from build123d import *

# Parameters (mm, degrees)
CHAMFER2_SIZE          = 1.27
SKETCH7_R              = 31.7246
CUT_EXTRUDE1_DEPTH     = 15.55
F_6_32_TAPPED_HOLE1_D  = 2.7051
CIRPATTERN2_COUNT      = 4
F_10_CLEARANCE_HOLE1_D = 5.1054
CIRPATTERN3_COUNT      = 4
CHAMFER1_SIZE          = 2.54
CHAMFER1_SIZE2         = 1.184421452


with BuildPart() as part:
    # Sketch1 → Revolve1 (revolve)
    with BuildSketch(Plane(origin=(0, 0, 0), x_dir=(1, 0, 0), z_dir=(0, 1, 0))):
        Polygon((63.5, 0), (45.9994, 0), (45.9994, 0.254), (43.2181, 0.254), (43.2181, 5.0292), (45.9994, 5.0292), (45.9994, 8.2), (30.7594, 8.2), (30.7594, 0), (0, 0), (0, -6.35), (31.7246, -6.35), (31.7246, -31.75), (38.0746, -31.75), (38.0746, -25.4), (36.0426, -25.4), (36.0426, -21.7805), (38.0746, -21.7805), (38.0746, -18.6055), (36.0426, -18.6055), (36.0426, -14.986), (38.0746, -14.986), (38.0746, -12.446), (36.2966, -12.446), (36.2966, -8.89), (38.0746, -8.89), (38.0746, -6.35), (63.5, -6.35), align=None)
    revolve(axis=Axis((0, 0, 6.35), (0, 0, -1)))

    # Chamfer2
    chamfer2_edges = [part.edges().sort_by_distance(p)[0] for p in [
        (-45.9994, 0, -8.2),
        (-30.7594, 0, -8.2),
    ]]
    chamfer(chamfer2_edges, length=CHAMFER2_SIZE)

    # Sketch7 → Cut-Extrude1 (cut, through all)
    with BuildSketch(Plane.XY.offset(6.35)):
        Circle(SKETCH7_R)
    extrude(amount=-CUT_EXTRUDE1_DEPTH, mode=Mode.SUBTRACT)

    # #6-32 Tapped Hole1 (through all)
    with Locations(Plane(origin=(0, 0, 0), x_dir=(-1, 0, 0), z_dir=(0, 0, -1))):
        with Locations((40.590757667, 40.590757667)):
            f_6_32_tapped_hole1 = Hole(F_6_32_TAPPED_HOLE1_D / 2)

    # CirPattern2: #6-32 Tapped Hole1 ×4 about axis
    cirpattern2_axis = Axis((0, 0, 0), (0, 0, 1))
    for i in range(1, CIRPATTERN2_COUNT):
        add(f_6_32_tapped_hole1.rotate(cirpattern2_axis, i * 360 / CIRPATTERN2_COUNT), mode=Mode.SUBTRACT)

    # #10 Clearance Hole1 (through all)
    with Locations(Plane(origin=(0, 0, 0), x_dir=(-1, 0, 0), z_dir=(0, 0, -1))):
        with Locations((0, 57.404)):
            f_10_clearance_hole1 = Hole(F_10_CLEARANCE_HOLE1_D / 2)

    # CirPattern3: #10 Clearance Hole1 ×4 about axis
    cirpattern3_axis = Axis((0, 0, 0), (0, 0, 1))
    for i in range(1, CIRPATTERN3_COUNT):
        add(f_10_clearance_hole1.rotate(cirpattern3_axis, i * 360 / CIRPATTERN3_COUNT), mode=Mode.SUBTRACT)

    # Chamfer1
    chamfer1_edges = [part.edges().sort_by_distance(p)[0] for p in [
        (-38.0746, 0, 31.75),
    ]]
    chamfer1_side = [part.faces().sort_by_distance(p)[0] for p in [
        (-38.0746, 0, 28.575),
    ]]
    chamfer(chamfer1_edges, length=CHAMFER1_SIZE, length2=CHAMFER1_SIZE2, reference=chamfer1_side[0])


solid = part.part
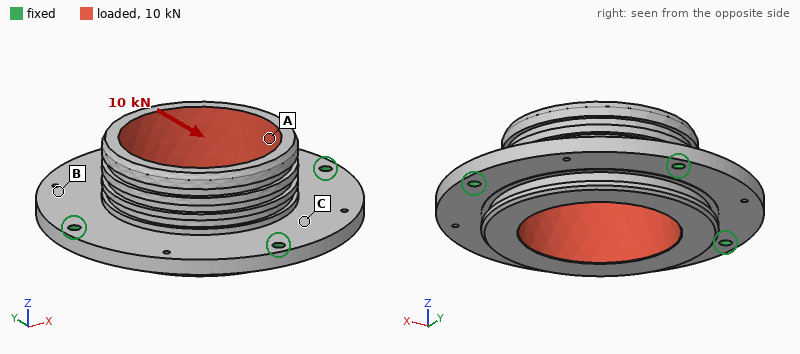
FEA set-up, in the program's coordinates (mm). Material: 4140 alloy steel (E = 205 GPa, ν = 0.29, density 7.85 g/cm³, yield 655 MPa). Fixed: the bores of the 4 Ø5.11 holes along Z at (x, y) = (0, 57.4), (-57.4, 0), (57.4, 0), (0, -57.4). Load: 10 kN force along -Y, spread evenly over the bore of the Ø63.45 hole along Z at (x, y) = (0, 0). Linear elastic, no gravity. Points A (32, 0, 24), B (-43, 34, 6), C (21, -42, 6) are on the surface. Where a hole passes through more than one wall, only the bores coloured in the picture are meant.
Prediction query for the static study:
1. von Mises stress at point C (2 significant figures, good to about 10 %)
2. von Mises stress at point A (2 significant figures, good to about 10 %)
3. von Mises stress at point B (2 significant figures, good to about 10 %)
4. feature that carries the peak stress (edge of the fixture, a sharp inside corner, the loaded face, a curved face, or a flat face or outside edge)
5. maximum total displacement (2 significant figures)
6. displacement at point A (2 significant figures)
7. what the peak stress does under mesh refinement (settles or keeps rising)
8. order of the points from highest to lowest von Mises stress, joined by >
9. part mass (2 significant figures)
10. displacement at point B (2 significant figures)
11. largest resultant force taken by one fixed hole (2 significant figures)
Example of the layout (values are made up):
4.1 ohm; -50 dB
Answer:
16 MPa; 9.2 MPa; 4.1 MPa; edge of the fixture; 11 µm; 8.0 µm; keeps rising; C > A > B; 900 g; 5.4 µm; 2.6 kN
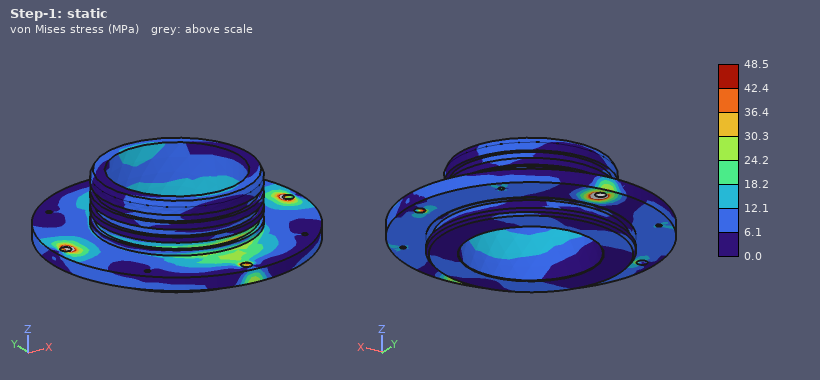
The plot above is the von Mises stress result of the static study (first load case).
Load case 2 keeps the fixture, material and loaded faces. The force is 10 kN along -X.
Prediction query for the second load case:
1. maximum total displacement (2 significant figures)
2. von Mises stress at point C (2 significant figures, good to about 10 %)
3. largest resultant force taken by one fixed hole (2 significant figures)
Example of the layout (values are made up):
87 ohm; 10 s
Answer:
11 µm; 7.2 MPa; 2.6 kN
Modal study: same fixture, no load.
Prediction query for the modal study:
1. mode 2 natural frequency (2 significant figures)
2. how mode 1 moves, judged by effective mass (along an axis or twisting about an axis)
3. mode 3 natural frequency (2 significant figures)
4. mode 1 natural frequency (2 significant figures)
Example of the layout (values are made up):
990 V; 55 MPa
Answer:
4600 Hz; along Z; 4700 Hz; 4400 Hz
